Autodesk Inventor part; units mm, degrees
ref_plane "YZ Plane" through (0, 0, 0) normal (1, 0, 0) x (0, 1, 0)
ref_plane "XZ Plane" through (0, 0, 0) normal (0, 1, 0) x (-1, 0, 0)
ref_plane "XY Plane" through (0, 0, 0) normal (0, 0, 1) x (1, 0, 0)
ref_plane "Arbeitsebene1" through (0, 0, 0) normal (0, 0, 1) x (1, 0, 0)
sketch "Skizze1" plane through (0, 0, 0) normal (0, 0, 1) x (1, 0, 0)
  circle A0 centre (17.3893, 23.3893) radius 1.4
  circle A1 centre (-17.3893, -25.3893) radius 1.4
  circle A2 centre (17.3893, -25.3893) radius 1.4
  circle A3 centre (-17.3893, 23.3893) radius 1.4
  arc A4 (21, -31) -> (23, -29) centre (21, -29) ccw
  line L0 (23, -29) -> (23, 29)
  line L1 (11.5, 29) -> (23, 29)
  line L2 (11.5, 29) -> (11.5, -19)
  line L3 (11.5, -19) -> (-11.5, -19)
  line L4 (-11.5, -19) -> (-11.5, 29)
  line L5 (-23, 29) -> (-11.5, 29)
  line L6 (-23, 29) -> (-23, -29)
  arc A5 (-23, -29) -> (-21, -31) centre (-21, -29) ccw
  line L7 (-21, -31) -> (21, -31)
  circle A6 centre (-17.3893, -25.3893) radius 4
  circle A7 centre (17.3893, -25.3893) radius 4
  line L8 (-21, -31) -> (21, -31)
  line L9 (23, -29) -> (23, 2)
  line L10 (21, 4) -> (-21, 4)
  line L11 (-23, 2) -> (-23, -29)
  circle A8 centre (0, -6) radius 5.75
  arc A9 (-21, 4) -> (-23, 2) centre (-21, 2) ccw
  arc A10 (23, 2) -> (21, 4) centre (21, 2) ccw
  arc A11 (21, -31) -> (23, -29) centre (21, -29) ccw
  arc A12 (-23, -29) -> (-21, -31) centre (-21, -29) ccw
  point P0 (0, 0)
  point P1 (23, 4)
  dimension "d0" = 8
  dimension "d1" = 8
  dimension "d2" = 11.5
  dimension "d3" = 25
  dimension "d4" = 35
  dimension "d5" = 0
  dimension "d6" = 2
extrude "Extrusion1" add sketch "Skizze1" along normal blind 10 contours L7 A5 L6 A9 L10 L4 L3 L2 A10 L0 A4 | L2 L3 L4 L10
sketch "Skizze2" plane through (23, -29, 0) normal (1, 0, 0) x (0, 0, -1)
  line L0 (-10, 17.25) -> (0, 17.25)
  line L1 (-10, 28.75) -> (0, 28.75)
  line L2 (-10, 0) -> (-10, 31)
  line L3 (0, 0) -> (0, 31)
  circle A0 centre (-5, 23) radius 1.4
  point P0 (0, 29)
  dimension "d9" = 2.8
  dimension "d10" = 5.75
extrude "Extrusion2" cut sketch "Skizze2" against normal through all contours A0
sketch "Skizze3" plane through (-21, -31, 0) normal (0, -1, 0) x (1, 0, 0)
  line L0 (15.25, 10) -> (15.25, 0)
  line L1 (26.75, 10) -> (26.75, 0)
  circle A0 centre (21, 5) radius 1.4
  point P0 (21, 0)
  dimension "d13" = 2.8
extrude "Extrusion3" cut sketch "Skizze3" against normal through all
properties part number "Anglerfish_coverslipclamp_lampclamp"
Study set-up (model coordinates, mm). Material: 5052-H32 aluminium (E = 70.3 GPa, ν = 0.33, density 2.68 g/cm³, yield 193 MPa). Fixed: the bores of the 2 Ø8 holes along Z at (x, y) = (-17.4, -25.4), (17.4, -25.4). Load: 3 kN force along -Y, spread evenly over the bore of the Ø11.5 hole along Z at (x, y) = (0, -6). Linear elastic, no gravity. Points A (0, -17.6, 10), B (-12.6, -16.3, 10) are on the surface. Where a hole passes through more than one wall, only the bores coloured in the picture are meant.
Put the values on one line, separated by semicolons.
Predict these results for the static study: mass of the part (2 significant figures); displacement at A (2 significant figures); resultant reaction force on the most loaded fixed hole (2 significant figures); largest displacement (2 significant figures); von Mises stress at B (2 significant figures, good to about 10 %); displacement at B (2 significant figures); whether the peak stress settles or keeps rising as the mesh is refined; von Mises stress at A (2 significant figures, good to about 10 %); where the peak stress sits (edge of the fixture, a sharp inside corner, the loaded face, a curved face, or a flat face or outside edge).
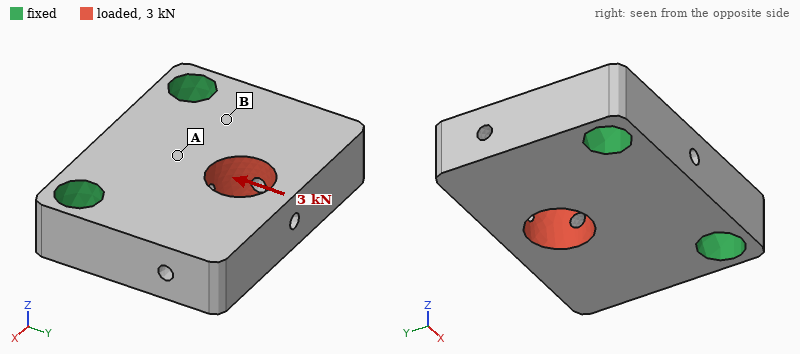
37 g; 2.7 µm; 1.6 kN; 7.3 µm; 12 MPa; 1.2 µm; keeps rising; 5.5 MPa; a sharp inside corner
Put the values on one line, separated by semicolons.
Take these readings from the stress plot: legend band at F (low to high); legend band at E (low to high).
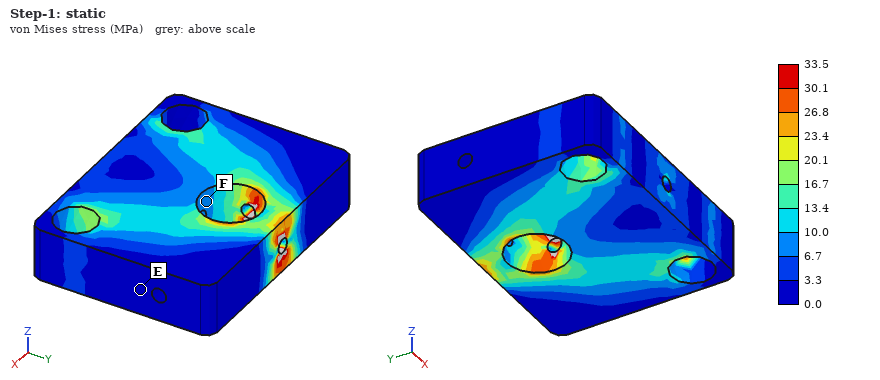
6.7 to 10.0 MPa; 0.0 to 3.3 MPa
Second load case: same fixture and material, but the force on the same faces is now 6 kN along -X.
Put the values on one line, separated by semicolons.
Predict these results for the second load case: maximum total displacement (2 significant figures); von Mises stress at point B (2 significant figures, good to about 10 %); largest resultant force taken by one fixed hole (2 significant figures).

22 µm; 25 MPa; 4.1 kN
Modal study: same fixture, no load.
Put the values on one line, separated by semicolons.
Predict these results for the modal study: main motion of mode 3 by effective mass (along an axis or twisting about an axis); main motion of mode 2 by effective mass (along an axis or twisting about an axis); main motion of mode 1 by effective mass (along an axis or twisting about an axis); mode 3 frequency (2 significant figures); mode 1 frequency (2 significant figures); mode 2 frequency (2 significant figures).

along X; twisting about Y; along Z; 21 kHz; 9400 Hz; 15 kHz
